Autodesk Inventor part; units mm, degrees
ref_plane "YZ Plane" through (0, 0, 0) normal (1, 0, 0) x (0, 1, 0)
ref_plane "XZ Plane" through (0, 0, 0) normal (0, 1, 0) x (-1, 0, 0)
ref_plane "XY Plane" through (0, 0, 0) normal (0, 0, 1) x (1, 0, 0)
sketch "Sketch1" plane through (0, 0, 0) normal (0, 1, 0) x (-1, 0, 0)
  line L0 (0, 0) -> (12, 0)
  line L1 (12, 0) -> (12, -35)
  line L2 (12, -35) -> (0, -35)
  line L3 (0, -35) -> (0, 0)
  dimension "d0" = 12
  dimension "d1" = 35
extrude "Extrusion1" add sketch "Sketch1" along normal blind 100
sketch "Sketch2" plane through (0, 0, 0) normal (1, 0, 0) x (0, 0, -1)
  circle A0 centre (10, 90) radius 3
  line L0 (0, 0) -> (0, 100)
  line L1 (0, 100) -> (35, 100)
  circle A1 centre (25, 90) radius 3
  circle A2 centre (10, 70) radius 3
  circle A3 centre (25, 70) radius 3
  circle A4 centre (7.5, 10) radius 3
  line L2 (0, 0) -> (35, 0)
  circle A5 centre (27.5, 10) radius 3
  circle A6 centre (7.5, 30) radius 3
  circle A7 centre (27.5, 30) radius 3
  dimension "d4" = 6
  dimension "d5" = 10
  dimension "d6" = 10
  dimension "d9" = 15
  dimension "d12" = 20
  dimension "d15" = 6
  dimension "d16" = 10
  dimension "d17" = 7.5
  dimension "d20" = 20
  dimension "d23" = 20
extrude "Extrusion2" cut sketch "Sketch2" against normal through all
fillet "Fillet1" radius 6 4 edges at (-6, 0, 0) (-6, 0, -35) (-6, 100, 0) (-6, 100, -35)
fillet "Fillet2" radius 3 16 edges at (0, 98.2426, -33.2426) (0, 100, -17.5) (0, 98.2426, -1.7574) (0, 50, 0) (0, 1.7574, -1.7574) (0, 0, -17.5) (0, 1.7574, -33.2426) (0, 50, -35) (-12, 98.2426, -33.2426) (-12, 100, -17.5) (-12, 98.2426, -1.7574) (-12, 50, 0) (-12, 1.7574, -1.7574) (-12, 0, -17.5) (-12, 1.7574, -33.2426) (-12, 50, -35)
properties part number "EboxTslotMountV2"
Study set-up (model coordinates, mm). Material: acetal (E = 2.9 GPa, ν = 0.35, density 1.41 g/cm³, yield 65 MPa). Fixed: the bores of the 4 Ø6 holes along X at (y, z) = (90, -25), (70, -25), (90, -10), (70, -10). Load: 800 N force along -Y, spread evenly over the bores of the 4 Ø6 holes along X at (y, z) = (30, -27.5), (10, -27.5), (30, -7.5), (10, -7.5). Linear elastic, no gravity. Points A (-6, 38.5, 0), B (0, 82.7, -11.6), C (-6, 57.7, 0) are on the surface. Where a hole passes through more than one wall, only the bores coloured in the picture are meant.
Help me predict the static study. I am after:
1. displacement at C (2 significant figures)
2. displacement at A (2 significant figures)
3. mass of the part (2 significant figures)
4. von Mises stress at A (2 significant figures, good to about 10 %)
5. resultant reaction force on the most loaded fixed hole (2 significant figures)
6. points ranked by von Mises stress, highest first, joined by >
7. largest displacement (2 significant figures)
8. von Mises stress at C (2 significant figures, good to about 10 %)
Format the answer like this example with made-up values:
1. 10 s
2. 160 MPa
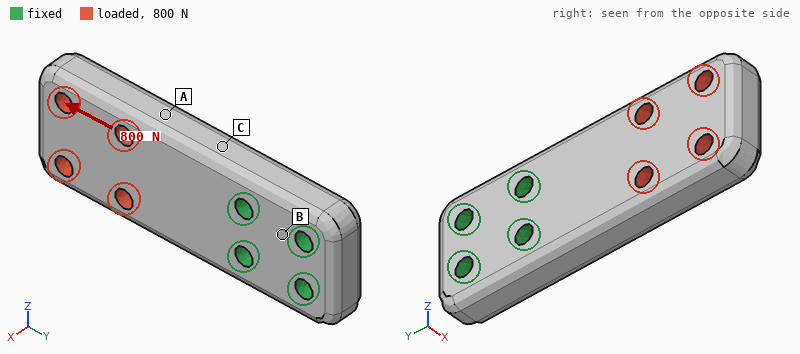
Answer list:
1. 10 µm
2. 22 µm
3. 53 g
4. 2.2 MPa
5. 370 N
6. A > C > B
7. 39 µm
8. 1.5 MPa
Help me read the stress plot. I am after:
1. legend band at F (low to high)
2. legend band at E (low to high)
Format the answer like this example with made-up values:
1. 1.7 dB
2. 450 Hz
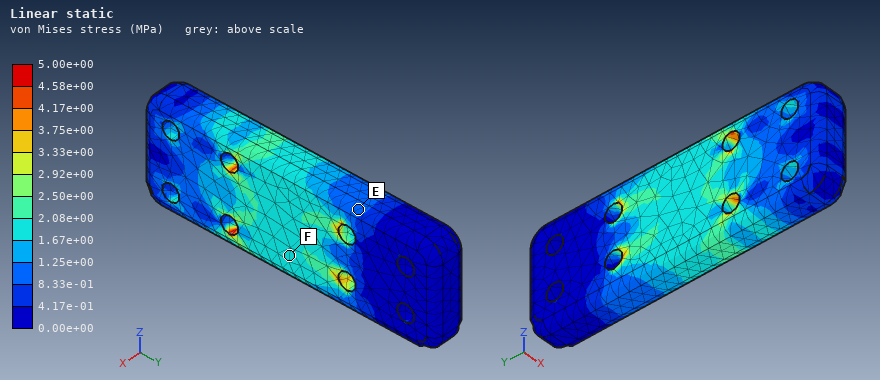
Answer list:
1. 1.67e+00 to 2.08e+00 MPa
2. 8.33e-01 to 1.25e+00 MPa
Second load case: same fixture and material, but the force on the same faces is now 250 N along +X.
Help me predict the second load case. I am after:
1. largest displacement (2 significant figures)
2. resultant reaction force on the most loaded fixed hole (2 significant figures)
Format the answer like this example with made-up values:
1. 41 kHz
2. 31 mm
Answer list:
1. 1.2 mm
2. 170 N
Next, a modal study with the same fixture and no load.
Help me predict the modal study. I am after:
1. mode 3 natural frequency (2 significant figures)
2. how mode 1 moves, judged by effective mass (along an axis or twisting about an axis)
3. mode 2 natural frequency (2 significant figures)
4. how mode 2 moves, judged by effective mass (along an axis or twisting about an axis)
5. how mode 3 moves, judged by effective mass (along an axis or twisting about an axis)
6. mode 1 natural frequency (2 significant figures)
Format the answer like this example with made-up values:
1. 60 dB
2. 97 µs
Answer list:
1. 2100 Hz
2. along X
3. 1400 Hz
4. along Z
5. twisting about Y
6. 600 Hz
